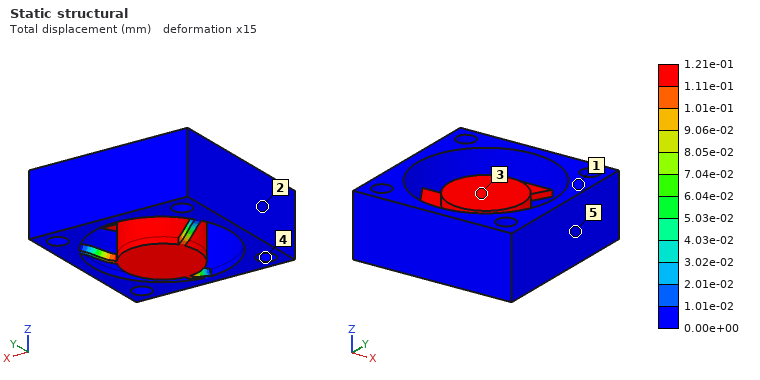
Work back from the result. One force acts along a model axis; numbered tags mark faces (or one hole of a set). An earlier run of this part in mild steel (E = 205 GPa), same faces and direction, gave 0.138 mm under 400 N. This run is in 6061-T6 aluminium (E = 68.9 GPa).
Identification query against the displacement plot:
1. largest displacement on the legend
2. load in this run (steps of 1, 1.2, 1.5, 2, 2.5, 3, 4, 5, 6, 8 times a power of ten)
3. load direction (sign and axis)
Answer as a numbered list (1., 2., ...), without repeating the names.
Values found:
1. 1.21e-01 mm
2. 120 N
3. -Z
